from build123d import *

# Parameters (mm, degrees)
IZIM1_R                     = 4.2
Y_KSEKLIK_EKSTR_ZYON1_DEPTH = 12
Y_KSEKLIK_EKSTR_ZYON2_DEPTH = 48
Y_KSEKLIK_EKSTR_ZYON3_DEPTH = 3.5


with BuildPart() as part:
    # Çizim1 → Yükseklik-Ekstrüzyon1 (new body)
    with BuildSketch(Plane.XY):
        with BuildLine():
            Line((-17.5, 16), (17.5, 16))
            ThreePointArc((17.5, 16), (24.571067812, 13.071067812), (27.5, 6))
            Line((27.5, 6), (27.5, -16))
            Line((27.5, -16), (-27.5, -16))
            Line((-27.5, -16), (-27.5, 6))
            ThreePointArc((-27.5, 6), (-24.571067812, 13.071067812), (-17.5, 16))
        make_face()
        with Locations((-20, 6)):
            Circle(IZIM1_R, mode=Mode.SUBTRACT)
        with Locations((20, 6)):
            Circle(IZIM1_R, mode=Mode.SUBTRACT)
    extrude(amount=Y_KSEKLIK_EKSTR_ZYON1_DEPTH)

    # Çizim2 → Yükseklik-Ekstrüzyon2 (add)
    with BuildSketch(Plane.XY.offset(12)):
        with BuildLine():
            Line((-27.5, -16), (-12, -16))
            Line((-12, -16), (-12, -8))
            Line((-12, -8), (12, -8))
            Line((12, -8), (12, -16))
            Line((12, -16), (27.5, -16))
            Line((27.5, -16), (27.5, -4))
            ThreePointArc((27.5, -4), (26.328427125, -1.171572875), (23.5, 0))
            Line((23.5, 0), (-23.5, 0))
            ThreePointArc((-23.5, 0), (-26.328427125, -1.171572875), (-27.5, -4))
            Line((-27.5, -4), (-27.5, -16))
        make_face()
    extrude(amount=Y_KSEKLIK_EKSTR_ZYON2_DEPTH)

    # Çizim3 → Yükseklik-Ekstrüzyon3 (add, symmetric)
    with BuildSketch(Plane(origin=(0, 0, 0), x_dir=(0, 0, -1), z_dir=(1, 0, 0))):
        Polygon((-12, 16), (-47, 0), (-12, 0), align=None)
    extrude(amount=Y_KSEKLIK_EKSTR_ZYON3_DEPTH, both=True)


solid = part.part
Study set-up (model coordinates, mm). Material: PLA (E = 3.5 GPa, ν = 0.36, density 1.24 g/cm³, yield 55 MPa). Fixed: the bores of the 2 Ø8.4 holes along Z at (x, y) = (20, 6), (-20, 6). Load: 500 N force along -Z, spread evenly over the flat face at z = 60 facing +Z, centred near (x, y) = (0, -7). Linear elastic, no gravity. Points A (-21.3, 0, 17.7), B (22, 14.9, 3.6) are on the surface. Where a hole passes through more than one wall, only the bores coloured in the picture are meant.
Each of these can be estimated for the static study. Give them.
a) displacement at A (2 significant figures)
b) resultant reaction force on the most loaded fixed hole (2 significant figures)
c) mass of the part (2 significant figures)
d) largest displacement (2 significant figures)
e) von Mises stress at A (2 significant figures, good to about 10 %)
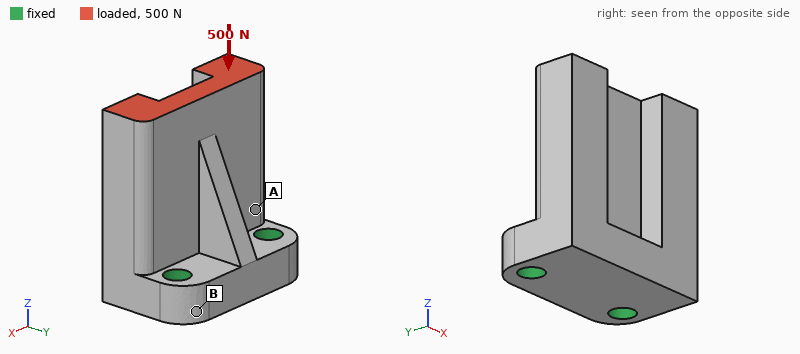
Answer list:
19 µm
250 N
67 g
96 µm
1.4 MPa
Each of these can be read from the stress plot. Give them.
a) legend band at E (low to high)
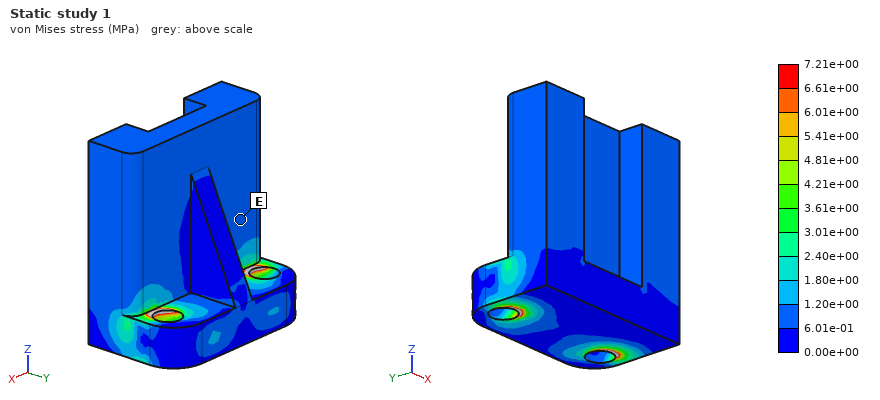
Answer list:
6.01e-01 to 1.20e+00 MPa
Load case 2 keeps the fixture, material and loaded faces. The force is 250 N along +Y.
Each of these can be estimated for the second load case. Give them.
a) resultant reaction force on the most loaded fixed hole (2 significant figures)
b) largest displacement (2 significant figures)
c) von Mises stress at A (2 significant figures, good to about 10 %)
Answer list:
130 N
0.41 mm
2.5 MPa
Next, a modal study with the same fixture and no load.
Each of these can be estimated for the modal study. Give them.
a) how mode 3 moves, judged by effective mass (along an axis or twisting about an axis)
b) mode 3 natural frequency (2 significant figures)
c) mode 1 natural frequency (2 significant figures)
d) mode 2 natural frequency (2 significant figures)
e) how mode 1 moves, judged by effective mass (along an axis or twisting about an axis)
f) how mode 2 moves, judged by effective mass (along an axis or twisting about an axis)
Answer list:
along X
2200 Hz
1100 Hz
2000 Hz
along Y
twisting about Z
